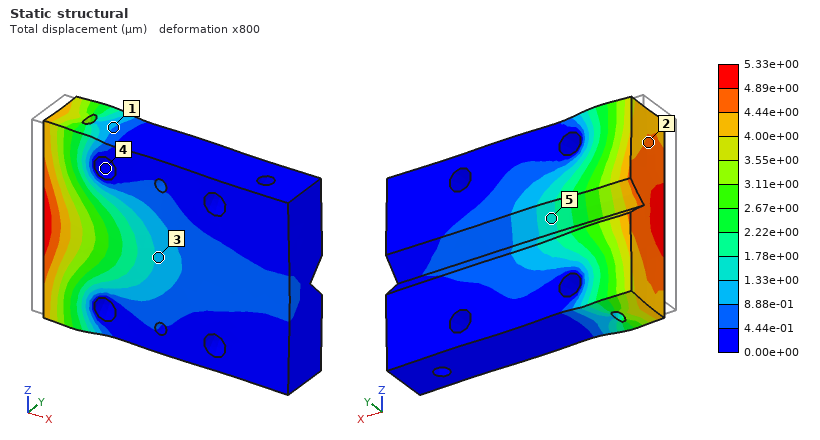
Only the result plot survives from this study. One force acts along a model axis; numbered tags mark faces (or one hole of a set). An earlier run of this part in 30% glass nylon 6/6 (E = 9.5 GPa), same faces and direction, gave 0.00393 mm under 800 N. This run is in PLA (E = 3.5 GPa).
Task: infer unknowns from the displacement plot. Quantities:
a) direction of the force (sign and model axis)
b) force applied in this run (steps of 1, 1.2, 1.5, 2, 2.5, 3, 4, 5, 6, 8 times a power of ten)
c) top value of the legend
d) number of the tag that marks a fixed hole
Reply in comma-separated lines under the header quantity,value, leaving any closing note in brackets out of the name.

quantity,value
direction of the force,+X
force applied in this run,400 N
top value of the legend,5.33e+00 µm
number of the tag that marks a fixed hole,4
